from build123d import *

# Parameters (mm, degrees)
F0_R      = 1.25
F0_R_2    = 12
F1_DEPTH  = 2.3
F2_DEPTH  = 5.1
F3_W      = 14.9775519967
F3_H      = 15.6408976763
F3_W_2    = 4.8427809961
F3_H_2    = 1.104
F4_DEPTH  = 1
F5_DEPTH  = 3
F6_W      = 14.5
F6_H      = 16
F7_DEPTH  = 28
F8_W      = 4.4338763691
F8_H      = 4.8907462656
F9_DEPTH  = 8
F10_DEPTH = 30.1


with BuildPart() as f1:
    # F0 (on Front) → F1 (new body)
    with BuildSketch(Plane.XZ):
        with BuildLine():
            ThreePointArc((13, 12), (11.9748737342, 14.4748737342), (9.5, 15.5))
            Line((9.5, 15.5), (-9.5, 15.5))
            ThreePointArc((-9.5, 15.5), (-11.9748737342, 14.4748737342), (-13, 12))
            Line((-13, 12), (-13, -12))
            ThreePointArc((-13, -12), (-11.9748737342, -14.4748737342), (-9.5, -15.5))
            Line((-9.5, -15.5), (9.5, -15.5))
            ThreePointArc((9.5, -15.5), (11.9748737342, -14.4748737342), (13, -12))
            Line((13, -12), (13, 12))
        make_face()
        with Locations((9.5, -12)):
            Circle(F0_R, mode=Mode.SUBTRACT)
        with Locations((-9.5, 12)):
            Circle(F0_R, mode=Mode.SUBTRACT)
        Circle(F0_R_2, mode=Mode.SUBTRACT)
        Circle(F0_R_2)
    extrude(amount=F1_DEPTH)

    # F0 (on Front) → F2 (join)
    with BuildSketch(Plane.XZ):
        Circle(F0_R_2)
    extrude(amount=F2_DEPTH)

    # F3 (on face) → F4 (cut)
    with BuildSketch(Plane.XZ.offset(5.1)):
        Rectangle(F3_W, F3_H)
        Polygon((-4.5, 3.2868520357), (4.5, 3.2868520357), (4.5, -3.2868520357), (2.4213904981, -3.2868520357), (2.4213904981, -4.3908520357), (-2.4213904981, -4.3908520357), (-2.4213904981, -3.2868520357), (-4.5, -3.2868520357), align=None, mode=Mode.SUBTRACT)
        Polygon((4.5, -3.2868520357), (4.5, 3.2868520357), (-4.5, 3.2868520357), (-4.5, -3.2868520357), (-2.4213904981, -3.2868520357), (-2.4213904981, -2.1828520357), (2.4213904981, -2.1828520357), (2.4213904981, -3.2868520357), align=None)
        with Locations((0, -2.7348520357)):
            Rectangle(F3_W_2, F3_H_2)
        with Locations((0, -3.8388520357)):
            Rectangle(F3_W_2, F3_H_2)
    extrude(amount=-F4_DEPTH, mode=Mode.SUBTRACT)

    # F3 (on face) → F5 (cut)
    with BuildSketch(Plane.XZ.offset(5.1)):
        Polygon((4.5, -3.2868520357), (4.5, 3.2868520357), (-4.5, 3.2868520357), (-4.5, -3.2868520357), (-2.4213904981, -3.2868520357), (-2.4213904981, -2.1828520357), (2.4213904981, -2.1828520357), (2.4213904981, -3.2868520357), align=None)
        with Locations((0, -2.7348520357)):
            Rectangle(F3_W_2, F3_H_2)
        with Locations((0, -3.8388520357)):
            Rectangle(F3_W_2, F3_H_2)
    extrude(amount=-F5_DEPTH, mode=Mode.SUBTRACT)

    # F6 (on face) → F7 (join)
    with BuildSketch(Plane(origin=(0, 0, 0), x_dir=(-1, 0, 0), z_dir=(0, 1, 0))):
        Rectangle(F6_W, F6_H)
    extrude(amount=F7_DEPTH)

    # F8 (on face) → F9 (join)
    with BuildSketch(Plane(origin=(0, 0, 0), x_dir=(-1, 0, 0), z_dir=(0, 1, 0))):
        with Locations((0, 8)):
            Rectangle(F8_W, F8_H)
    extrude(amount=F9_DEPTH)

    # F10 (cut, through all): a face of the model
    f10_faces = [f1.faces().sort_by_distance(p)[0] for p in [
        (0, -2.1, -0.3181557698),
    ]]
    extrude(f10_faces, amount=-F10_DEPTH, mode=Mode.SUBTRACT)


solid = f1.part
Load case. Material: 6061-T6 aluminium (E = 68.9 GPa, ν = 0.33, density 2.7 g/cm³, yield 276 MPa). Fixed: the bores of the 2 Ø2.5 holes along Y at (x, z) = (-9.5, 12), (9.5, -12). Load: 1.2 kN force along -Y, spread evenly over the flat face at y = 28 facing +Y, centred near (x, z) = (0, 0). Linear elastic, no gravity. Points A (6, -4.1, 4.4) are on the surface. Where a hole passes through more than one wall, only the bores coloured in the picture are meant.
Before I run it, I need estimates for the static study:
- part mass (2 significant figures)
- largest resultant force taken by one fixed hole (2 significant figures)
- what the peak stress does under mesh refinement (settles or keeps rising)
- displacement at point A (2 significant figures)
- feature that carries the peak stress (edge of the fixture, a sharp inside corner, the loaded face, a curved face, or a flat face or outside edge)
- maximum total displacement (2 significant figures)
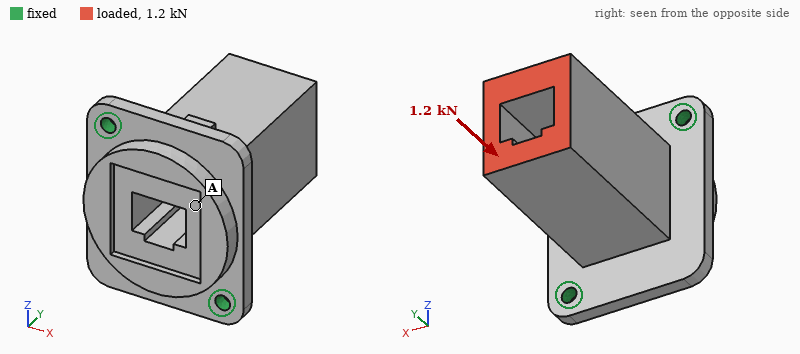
20 g
600 N
keeps rising
22 µm
edge of the fixture
27 µm
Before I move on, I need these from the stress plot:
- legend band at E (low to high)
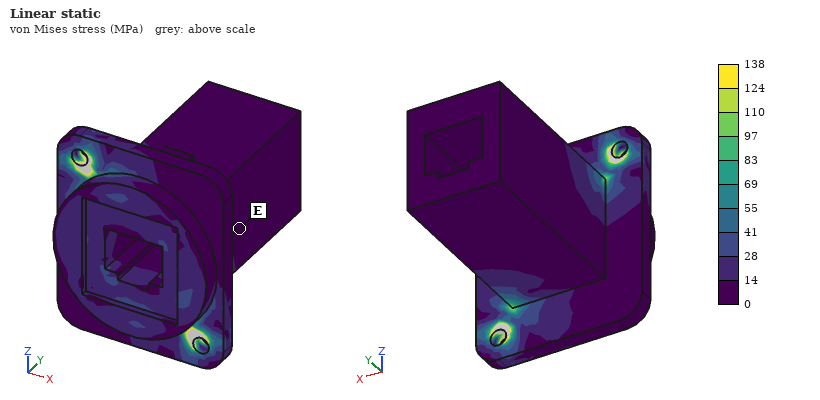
0 to 14 MPa
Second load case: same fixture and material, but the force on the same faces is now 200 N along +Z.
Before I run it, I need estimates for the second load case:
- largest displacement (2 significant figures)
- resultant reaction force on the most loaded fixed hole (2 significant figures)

0.19 mm
200 N
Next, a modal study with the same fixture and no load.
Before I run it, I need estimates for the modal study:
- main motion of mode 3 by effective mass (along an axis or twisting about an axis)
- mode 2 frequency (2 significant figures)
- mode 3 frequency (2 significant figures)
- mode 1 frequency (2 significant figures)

along Y
6900 Hz
8700 Hz
1800 Hz
